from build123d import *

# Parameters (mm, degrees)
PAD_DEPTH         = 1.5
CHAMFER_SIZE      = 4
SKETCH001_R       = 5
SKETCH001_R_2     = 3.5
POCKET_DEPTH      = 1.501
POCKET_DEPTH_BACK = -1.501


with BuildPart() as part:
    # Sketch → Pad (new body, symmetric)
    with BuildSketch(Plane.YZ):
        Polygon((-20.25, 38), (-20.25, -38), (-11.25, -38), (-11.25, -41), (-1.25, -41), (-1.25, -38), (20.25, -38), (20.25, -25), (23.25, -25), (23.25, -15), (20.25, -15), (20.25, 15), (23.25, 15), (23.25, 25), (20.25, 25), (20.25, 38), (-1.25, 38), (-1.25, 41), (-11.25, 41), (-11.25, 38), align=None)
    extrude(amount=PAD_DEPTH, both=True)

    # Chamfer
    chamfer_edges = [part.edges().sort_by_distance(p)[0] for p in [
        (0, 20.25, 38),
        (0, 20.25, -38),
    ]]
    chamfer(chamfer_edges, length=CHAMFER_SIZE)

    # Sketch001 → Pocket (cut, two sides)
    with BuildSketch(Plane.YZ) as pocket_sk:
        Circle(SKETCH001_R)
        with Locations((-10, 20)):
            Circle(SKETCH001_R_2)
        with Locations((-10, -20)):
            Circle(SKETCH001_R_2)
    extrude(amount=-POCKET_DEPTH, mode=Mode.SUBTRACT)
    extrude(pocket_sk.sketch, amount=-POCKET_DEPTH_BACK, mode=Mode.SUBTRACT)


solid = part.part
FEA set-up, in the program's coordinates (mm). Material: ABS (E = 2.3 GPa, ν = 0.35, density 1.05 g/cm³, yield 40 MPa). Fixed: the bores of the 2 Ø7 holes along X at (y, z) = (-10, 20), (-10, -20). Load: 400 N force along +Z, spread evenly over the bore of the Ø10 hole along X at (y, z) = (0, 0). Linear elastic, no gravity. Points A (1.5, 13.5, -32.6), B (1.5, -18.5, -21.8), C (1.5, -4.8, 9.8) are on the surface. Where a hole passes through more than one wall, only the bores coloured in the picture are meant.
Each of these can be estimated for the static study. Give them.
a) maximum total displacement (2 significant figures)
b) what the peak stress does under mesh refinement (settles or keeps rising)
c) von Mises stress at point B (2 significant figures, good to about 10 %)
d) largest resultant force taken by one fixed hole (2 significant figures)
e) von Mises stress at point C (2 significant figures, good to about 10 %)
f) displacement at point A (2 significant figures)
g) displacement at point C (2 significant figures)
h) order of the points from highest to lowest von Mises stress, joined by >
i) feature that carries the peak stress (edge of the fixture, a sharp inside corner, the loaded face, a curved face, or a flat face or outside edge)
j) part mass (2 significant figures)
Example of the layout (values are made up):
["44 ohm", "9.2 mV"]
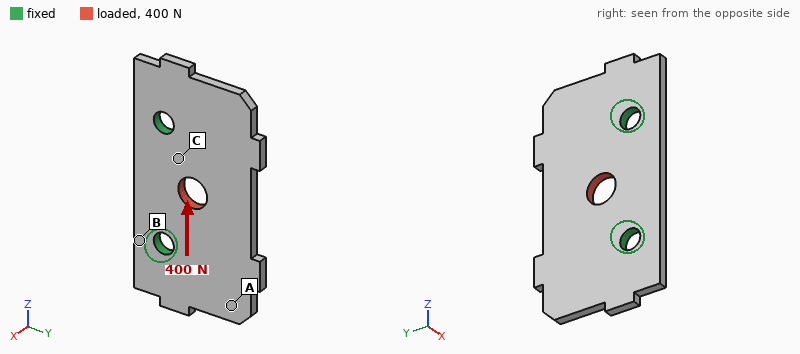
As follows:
["58 µm", "keeps rising", "1.5 MPa", "220 N", "4.6 MPa", "45 µm", "20 µm", "C > B > A", "edge of the fixture", "9.5 g"]
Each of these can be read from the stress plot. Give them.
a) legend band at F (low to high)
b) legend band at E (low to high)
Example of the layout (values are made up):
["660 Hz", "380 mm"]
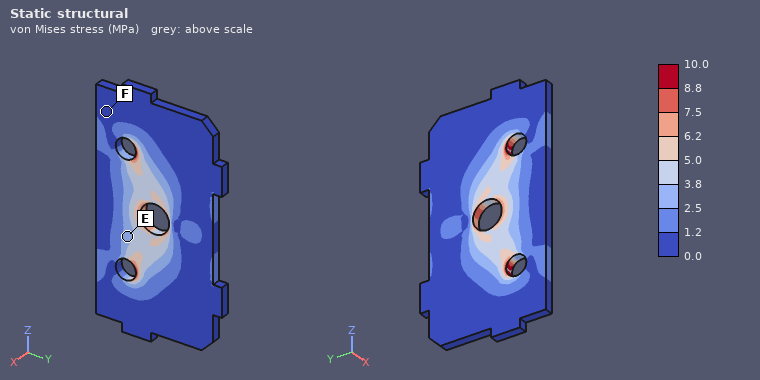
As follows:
["0.0 to 1.2 MPa", "2.5 to 3.8 MPa"]
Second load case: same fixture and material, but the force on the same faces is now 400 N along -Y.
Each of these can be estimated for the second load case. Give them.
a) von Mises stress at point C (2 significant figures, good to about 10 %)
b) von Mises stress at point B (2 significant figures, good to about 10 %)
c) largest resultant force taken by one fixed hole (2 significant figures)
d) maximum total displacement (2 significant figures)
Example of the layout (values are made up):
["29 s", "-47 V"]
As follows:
["3.9 MPa", "1.4 MPa", "210 N", "56 µm"]
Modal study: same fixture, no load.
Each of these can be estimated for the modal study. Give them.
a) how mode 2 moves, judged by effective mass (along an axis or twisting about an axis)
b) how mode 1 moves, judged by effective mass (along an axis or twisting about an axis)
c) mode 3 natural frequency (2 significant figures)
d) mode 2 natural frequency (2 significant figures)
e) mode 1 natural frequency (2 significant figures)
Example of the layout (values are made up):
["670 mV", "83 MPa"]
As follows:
["twisting about Y", "along X", "1500 Hz", "1000 Hz", "770 Hz"]
